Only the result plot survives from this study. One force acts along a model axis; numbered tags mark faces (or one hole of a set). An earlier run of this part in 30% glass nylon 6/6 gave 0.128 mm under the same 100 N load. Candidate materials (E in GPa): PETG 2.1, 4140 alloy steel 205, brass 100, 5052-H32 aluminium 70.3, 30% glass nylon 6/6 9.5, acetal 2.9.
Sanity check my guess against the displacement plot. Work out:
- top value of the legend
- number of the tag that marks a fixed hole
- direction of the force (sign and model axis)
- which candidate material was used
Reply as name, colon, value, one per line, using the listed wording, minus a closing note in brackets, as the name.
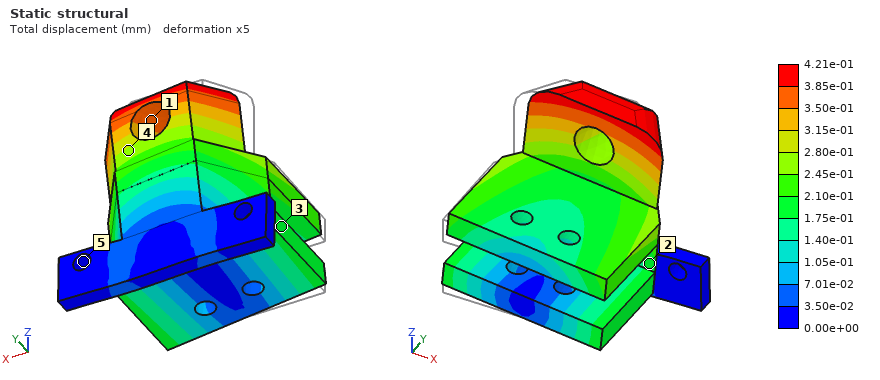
top value of the legend: 4.21e-01 mm
number of the tag that marks a fixed hole: 5
direction of the force: +X
which candidate material was used: acetal
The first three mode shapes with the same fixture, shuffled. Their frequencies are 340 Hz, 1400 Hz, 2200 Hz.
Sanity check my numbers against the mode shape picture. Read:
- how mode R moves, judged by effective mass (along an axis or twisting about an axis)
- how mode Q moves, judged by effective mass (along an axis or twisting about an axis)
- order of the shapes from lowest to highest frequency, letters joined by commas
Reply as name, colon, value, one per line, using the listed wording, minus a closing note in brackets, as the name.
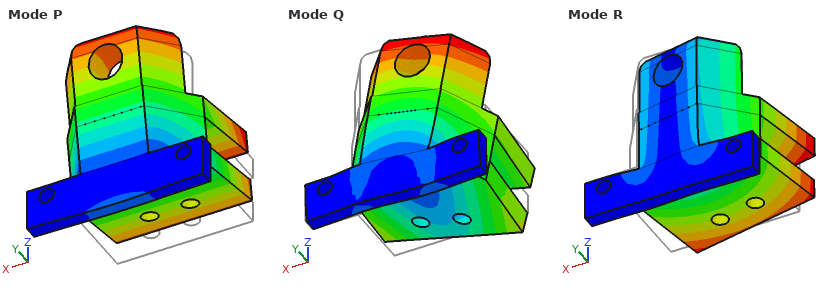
how mode R moves, judged by effective mass: along X
how mode Q moves, judged by effective mass: along X
order of the shapes from lowest to highest frequency, letters joined by commas: P, R, Q
